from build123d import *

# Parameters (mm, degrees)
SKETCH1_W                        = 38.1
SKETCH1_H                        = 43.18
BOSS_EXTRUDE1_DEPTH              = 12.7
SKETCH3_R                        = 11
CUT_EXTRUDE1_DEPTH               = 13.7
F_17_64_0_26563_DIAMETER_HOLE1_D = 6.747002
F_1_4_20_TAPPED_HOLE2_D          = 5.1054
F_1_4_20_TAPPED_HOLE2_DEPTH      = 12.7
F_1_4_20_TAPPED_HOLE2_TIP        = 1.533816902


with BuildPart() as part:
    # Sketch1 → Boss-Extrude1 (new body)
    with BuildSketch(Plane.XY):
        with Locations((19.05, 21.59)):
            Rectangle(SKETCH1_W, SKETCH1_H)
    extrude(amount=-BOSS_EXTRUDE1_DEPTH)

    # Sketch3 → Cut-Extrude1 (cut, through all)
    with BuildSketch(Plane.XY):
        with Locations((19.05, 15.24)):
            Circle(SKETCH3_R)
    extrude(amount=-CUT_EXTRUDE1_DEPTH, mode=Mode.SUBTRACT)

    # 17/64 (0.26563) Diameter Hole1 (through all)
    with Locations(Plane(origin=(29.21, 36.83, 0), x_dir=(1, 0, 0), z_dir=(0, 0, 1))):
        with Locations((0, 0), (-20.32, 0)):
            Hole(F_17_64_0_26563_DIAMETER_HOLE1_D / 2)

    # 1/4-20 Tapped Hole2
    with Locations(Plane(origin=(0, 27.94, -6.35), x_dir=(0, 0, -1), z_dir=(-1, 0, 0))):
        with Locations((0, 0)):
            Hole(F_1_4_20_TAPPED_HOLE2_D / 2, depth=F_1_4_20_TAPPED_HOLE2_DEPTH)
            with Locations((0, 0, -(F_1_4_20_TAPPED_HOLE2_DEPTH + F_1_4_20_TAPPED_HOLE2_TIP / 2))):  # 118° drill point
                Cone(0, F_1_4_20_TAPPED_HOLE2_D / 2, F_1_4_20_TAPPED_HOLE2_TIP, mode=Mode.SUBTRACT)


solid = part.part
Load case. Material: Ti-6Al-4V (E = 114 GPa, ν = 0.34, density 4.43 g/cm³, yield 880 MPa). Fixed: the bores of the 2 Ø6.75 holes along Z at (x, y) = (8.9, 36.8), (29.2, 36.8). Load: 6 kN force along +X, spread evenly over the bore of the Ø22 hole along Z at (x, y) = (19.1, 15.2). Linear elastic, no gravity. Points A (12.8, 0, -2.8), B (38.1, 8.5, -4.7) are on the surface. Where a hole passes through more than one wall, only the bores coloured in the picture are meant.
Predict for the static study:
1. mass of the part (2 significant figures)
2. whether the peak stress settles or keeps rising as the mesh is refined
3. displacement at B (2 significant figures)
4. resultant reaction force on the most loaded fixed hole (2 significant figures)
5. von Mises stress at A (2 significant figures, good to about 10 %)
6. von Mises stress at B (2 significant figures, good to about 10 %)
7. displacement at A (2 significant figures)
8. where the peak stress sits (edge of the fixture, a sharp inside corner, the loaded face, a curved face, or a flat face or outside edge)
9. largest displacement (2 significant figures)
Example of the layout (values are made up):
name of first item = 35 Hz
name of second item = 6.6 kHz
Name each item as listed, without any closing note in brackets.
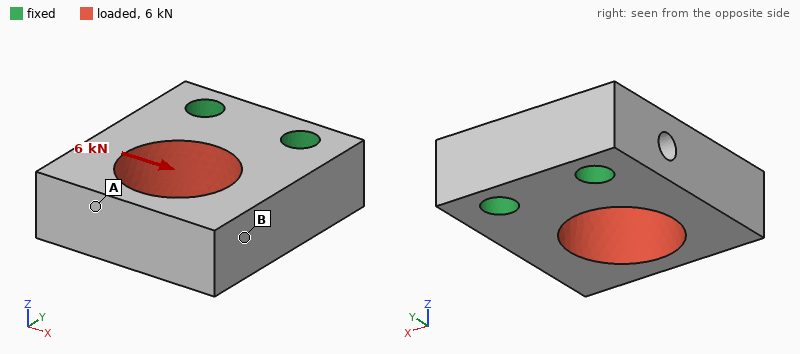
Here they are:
mass of the part = 66 g
whether the peak stress settles or keeps rising as the mesh is refined = keeps rising
displacement at B = 41 µm
resultant reaction force on the most loaded fixed hole = 5.1 kN
von Mises stress at A = 62 MPa
von Mises stress at B = 26 MPa
displacement at A = 47 µm
where the peak stress sits = a sharp inside corner
largest displacement = 52 µm
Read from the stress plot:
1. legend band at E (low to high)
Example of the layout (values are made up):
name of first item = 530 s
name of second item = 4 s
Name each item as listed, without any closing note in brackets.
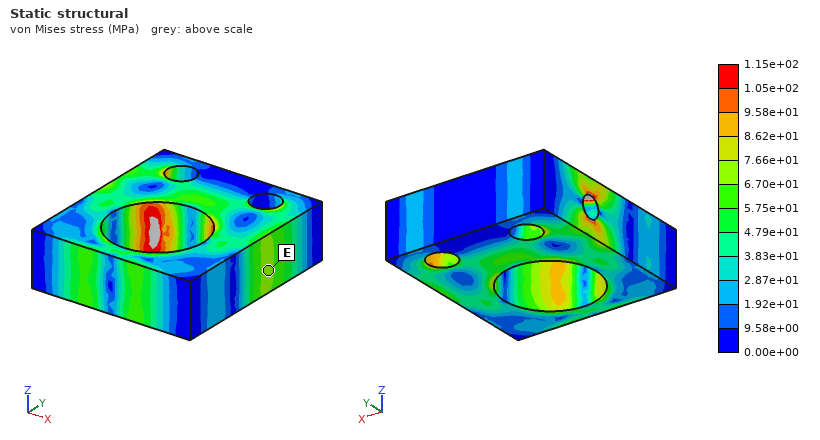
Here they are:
legend band at E = 6.70e+01 to 7.66e+01 MPa
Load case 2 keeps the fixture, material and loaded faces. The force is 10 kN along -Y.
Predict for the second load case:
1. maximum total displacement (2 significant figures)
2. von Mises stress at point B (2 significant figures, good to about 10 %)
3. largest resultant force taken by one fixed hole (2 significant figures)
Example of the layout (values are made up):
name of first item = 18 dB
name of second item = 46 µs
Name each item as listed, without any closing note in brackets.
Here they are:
maximum total displacement = 23 µm
von Mises stress at point B = 19 MPa
largest resultant force taken by one fixed hole = 5.0 kN
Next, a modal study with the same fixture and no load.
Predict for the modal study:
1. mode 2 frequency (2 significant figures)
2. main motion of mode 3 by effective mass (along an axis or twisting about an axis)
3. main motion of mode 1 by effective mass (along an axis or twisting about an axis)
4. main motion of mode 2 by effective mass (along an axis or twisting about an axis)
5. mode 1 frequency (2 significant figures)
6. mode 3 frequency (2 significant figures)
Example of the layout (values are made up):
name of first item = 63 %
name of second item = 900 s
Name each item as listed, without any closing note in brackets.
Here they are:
mode 2 frequency = 9300 Hz
main motion of mode 3 by effective mass = twisting about Y
main motion of mode 1 by effective mass = along Z
main motion of mode 2 by effective mass = along X
mode 1 frequency = 6900 Hz
mode 3 frequency = 11 kHz
